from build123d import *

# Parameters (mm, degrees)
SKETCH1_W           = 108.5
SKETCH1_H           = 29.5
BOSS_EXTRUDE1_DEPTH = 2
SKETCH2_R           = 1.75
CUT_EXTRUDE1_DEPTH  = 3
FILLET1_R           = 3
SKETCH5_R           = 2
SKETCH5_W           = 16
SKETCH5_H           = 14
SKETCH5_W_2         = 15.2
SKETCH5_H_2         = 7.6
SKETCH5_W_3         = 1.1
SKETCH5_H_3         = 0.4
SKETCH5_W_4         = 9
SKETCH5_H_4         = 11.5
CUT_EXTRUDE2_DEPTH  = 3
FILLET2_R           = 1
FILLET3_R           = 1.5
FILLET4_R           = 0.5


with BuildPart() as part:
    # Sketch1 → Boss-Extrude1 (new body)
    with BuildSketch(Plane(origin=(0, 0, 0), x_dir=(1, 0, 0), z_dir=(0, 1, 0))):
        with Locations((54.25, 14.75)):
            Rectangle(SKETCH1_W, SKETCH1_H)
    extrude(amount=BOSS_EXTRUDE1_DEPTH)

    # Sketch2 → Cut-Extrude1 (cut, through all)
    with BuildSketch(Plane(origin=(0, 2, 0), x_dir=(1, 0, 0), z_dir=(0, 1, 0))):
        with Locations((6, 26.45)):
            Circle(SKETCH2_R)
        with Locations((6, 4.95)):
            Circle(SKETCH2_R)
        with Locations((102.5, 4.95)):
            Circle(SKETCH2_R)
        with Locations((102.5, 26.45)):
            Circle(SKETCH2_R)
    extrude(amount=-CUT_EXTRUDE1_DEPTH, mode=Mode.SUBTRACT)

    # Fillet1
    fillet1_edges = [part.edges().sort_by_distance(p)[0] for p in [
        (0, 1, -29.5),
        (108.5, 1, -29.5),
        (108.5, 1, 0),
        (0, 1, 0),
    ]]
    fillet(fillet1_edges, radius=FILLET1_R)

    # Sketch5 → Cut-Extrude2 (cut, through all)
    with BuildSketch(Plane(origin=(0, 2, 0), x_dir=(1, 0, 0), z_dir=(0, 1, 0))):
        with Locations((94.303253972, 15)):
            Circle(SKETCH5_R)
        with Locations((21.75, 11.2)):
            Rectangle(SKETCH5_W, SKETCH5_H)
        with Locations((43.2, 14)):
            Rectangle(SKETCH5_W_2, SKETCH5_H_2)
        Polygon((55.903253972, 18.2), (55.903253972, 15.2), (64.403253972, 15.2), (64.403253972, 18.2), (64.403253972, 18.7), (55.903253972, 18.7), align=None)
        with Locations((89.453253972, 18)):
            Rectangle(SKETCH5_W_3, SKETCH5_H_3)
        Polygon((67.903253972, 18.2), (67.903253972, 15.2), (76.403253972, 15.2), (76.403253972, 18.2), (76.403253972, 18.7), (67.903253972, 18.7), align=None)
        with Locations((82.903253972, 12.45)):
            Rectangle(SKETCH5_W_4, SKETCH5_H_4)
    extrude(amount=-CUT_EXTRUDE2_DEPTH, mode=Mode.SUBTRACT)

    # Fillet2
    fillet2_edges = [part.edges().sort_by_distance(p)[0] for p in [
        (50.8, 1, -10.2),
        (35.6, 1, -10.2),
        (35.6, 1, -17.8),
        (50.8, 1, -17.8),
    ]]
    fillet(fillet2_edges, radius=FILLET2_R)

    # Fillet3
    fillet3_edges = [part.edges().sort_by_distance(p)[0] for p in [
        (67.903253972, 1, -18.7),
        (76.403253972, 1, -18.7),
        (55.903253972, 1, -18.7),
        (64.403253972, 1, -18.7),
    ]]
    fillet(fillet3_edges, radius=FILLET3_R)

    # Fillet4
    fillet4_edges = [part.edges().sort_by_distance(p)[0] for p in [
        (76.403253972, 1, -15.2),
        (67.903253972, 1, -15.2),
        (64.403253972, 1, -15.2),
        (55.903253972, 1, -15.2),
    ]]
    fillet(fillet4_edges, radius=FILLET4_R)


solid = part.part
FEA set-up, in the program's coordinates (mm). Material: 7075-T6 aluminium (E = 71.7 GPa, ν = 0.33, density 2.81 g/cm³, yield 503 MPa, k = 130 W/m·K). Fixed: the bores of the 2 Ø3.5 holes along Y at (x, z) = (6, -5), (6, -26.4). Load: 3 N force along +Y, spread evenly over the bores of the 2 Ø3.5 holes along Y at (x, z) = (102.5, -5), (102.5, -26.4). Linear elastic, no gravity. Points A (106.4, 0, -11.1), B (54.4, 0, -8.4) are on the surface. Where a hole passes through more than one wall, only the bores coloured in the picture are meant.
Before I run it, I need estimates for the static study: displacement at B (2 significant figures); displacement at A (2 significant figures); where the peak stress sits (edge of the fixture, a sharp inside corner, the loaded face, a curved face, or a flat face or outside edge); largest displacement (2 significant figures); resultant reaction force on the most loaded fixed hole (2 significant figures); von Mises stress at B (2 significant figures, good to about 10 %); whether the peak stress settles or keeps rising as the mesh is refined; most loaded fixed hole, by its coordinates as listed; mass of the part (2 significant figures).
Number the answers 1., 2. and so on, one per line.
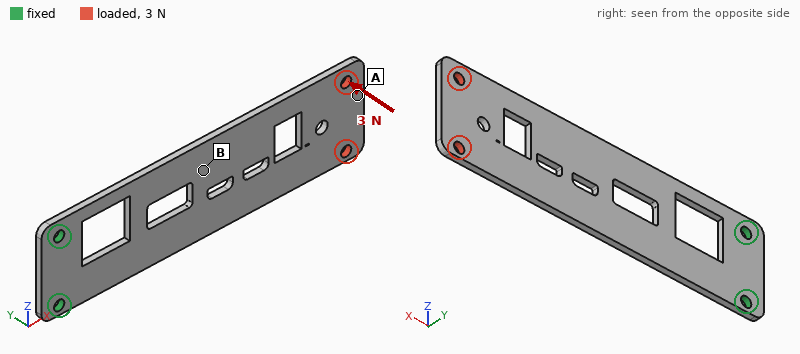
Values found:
1. 0.32 mm
2. 1.0 mm
3. edge of the fixture
4. 1.1 mm
5. 2.1 N
6. 7.9 MPa
7. keeps rising
8. (6, -26.4)
9. 15 g
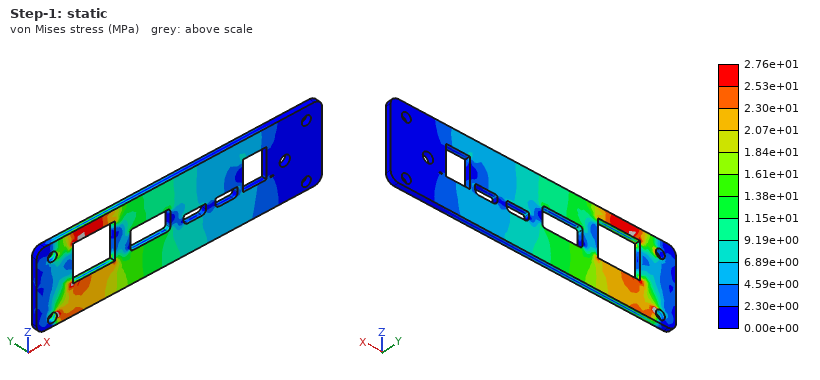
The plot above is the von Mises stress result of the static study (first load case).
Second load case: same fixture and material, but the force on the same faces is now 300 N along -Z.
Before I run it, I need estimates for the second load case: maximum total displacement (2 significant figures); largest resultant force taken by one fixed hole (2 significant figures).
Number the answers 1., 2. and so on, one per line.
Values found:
1. 0.48 mm
2. 1.3 kN
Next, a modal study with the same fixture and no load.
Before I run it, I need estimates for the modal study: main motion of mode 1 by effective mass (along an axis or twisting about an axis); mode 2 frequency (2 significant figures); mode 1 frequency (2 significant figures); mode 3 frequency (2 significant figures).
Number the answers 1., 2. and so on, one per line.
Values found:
1. along Y
2. 910 Hz
3. 130 Hz
4. 950 Hz
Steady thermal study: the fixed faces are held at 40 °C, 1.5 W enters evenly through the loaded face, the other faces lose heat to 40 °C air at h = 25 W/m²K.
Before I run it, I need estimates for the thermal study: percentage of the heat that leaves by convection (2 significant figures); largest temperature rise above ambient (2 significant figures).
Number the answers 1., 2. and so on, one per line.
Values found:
1. 65 %
2. 15 K
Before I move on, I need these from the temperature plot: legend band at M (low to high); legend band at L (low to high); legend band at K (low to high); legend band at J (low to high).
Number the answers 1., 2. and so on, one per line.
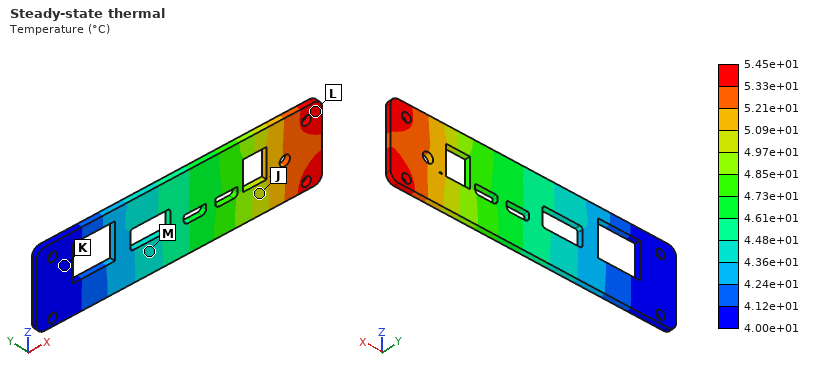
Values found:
1. 4.36e+01 to 4.48e+01 °C
2. 5.33e+01 to 5.45e+01 °C
3. 4.00e+01 to 4.12e+01 °C
4. 4.97e+01 to 5.09e+01 °C
